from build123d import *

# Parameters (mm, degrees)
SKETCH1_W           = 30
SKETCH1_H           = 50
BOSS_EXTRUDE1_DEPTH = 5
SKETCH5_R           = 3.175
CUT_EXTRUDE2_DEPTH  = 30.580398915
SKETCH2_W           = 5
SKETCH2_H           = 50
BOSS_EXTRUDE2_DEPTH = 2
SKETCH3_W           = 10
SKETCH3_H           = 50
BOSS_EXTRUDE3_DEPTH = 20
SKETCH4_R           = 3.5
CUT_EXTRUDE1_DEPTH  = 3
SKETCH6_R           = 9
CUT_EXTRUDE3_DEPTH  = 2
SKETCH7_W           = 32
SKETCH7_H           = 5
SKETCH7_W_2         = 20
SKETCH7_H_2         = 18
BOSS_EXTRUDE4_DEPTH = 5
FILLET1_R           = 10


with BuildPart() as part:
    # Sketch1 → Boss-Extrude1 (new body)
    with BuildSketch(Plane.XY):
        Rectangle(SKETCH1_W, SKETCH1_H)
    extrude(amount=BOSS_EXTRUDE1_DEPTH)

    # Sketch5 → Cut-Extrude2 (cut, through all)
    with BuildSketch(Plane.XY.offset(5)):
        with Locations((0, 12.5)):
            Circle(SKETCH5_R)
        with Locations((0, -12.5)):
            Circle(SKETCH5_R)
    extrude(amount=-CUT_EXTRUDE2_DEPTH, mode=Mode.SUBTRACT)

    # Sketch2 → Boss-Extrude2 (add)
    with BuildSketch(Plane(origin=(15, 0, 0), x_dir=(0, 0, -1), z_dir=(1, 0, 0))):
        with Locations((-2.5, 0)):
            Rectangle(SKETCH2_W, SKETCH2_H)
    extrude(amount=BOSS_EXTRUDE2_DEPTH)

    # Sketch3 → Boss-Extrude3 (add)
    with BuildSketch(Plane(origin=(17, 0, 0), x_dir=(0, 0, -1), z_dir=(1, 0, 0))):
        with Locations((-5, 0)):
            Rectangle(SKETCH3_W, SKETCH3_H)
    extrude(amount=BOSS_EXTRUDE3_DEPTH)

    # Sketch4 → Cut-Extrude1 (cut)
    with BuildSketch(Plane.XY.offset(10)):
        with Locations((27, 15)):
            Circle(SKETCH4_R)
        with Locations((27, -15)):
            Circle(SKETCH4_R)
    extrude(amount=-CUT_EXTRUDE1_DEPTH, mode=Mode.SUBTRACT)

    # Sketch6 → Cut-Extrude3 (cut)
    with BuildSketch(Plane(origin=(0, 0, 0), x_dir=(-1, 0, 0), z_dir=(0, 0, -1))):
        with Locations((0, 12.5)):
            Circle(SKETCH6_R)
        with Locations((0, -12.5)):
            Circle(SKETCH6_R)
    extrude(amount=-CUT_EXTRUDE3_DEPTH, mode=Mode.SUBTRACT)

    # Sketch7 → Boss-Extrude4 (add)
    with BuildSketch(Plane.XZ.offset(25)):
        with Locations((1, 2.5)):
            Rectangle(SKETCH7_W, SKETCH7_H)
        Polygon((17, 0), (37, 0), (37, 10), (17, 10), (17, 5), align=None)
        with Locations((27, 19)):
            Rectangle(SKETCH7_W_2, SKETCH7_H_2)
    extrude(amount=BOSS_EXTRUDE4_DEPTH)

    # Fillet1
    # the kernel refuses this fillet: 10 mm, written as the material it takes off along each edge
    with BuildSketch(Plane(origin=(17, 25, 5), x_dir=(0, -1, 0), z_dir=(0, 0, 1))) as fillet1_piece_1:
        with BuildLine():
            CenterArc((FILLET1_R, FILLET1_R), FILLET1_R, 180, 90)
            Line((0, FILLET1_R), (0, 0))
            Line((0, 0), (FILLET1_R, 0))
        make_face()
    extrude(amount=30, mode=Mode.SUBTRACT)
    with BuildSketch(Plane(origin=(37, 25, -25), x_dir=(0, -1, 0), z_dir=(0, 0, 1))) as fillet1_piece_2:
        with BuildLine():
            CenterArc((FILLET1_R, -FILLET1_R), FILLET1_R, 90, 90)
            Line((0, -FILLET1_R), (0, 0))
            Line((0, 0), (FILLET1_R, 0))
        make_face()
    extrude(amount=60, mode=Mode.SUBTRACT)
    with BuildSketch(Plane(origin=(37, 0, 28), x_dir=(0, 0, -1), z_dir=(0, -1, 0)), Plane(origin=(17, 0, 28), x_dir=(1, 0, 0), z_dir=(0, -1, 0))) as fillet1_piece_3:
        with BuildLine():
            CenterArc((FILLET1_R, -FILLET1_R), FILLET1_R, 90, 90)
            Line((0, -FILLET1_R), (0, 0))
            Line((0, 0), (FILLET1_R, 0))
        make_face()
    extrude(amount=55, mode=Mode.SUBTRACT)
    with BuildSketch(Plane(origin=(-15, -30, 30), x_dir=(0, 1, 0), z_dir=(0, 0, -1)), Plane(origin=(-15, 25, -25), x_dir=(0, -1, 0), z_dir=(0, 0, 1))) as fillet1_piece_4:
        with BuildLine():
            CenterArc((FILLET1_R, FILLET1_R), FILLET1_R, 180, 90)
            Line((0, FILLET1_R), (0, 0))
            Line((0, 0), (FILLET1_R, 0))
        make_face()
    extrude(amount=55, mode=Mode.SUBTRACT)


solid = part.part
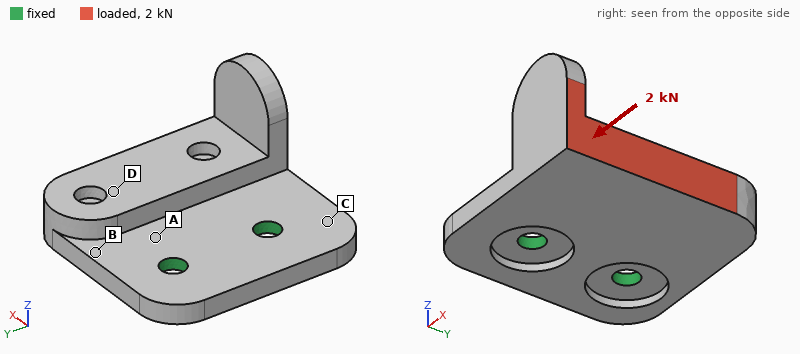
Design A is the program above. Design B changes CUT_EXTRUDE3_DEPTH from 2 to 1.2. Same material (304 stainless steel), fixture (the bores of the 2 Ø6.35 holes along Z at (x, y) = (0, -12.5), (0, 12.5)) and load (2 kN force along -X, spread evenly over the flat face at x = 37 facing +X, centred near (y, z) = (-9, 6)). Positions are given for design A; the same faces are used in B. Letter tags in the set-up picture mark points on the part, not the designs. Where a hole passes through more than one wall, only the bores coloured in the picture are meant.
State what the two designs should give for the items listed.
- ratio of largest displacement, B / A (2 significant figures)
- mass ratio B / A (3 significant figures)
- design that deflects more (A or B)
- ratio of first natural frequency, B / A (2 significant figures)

0.89
1.02
A
1.2
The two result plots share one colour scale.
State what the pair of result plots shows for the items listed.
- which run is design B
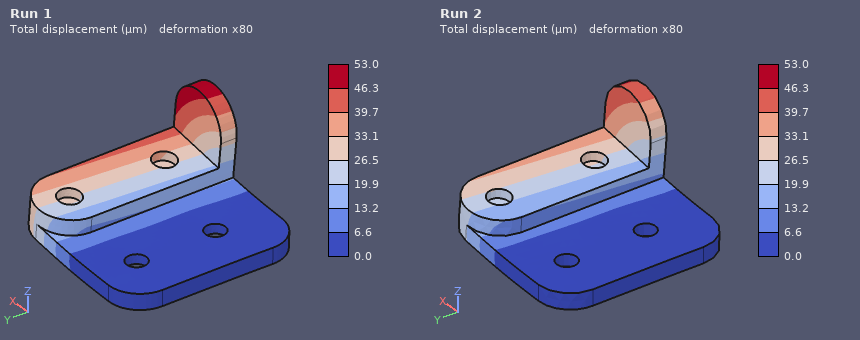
Run 2
